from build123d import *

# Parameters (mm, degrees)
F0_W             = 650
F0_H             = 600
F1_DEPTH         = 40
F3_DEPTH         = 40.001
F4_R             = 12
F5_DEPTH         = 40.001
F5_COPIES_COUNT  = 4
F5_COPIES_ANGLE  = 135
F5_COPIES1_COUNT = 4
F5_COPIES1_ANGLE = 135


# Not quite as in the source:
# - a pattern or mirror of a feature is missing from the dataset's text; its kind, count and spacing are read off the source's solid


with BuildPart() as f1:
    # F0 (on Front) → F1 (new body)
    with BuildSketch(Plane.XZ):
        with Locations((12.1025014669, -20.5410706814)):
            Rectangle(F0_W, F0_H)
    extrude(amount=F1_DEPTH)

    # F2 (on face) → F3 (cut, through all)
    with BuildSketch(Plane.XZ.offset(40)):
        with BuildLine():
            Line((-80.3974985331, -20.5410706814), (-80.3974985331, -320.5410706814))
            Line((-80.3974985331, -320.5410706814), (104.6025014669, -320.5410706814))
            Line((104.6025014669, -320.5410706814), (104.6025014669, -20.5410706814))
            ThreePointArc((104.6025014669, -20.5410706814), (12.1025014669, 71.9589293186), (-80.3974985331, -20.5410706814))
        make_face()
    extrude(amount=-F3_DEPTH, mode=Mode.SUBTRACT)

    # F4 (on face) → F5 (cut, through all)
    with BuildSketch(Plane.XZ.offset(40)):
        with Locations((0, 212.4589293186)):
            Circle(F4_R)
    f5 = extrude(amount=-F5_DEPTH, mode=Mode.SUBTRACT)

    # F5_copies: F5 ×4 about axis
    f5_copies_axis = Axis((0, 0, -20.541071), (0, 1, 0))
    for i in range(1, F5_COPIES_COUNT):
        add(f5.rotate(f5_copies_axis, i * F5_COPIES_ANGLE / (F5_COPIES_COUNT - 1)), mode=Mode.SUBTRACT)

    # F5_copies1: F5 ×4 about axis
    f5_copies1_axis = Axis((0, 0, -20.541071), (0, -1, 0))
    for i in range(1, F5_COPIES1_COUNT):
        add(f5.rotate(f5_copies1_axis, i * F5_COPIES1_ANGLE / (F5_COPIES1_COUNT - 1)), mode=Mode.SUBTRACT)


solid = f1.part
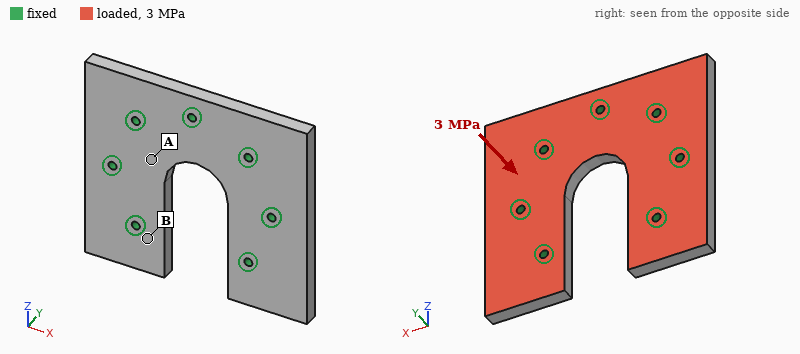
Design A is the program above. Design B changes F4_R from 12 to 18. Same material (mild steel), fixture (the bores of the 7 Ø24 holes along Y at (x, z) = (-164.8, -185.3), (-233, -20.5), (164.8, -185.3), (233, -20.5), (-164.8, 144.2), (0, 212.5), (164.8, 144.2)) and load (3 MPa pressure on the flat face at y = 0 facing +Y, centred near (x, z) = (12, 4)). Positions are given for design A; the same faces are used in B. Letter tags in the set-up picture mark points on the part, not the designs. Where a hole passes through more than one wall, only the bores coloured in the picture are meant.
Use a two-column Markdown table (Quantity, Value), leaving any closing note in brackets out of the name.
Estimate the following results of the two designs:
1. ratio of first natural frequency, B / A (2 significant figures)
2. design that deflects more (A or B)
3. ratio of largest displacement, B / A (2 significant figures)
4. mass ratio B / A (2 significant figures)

| Quantity | Value |
|---|---|
| ratio of first natural frequency, B / A | 1.1 |
| design that deflects more | A |
| ratio of largest displacement, B / A | 0.82 |
| mass ratio B / A | 0.99 |
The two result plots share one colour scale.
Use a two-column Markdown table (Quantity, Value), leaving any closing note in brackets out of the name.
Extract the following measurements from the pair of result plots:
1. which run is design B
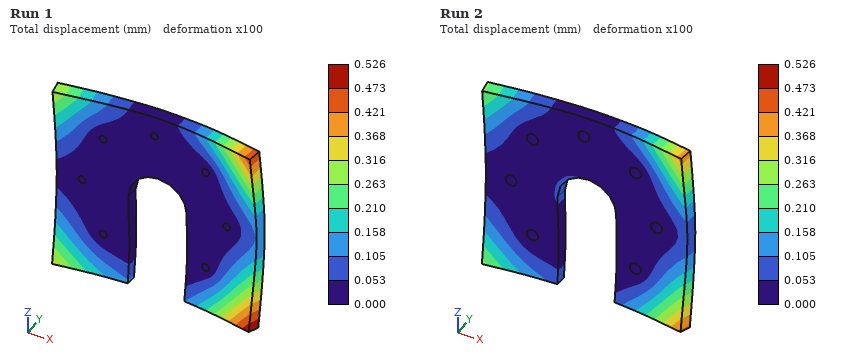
| Quantity | Value |
|---|---|
| which run is design B | Run 2 |
